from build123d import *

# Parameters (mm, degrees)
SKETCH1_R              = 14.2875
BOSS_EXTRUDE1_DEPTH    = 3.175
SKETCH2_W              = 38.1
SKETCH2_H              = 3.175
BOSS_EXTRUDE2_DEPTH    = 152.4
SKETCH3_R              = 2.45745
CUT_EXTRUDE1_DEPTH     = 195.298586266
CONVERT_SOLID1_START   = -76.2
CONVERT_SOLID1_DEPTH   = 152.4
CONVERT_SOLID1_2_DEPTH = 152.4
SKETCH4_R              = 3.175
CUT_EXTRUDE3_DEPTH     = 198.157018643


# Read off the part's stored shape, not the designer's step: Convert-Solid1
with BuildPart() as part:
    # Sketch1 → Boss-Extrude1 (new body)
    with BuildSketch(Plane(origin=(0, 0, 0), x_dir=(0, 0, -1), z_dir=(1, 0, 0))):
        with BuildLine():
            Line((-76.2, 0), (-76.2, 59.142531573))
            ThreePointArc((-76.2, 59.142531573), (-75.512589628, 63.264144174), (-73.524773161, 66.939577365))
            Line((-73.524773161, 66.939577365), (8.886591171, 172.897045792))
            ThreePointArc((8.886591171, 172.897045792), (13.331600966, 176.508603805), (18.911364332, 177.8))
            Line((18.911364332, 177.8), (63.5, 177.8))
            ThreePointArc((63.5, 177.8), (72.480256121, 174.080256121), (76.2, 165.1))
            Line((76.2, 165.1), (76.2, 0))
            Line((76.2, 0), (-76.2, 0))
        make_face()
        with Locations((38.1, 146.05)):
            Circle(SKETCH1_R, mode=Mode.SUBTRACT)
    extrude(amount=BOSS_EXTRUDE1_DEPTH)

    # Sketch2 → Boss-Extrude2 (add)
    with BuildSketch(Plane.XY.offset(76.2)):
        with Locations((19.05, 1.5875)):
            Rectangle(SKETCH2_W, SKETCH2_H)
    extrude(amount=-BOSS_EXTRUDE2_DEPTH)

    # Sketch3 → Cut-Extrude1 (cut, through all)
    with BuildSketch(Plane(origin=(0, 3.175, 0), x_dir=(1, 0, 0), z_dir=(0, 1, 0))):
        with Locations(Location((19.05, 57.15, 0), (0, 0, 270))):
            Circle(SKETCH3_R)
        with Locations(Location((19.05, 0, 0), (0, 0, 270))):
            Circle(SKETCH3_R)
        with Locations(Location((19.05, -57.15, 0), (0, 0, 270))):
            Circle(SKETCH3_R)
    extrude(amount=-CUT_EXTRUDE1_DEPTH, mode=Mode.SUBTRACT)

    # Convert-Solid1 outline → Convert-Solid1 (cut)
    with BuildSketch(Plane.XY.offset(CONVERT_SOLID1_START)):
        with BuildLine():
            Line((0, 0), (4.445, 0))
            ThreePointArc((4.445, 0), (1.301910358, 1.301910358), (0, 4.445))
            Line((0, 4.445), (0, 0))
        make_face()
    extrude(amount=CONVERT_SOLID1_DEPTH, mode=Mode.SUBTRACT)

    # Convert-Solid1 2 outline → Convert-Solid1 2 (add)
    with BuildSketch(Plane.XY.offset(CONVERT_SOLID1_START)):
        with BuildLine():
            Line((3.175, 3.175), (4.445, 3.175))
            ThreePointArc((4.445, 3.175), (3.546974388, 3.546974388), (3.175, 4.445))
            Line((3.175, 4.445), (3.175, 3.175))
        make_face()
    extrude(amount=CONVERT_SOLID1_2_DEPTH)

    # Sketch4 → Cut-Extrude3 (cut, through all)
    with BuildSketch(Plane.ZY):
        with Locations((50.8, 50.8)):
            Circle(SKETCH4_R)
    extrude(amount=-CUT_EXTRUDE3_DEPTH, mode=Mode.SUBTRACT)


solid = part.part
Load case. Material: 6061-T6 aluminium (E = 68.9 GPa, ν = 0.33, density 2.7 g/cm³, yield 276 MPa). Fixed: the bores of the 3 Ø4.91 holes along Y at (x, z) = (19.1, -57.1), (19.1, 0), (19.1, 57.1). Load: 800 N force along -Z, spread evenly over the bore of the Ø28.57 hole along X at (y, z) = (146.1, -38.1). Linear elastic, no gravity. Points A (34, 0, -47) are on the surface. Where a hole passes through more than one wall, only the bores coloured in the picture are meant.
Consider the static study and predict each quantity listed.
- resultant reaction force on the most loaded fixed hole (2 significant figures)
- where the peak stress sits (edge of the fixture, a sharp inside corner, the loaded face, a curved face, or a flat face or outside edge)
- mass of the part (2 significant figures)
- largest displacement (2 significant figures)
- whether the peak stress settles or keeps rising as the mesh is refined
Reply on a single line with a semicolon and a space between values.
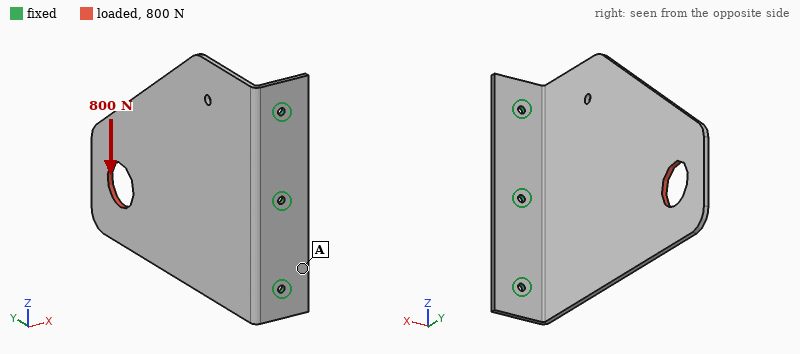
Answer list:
1.0 kN; edge of the fixture; 230 g; 1.0 mm; keeps rising
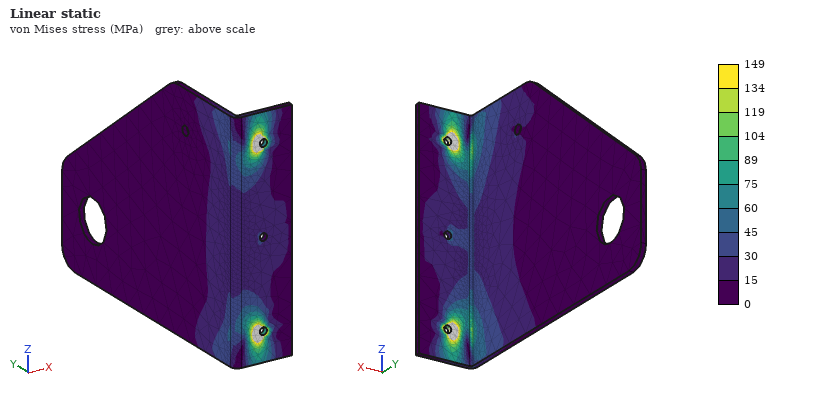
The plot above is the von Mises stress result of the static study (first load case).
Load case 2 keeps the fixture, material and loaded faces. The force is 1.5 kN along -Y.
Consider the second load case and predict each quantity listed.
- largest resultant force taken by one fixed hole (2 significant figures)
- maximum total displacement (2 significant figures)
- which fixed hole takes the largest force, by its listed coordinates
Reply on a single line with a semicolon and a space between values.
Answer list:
980 N; 2.1 mm; (19.1, -57.1)
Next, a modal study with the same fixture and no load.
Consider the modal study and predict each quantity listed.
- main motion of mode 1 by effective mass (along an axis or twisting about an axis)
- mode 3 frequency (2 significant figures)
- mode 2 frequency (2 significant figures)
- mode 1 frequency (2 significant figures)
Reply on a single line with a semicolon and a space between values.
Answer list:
along X; 500 Hz; 330 Hz; 94 Hz
